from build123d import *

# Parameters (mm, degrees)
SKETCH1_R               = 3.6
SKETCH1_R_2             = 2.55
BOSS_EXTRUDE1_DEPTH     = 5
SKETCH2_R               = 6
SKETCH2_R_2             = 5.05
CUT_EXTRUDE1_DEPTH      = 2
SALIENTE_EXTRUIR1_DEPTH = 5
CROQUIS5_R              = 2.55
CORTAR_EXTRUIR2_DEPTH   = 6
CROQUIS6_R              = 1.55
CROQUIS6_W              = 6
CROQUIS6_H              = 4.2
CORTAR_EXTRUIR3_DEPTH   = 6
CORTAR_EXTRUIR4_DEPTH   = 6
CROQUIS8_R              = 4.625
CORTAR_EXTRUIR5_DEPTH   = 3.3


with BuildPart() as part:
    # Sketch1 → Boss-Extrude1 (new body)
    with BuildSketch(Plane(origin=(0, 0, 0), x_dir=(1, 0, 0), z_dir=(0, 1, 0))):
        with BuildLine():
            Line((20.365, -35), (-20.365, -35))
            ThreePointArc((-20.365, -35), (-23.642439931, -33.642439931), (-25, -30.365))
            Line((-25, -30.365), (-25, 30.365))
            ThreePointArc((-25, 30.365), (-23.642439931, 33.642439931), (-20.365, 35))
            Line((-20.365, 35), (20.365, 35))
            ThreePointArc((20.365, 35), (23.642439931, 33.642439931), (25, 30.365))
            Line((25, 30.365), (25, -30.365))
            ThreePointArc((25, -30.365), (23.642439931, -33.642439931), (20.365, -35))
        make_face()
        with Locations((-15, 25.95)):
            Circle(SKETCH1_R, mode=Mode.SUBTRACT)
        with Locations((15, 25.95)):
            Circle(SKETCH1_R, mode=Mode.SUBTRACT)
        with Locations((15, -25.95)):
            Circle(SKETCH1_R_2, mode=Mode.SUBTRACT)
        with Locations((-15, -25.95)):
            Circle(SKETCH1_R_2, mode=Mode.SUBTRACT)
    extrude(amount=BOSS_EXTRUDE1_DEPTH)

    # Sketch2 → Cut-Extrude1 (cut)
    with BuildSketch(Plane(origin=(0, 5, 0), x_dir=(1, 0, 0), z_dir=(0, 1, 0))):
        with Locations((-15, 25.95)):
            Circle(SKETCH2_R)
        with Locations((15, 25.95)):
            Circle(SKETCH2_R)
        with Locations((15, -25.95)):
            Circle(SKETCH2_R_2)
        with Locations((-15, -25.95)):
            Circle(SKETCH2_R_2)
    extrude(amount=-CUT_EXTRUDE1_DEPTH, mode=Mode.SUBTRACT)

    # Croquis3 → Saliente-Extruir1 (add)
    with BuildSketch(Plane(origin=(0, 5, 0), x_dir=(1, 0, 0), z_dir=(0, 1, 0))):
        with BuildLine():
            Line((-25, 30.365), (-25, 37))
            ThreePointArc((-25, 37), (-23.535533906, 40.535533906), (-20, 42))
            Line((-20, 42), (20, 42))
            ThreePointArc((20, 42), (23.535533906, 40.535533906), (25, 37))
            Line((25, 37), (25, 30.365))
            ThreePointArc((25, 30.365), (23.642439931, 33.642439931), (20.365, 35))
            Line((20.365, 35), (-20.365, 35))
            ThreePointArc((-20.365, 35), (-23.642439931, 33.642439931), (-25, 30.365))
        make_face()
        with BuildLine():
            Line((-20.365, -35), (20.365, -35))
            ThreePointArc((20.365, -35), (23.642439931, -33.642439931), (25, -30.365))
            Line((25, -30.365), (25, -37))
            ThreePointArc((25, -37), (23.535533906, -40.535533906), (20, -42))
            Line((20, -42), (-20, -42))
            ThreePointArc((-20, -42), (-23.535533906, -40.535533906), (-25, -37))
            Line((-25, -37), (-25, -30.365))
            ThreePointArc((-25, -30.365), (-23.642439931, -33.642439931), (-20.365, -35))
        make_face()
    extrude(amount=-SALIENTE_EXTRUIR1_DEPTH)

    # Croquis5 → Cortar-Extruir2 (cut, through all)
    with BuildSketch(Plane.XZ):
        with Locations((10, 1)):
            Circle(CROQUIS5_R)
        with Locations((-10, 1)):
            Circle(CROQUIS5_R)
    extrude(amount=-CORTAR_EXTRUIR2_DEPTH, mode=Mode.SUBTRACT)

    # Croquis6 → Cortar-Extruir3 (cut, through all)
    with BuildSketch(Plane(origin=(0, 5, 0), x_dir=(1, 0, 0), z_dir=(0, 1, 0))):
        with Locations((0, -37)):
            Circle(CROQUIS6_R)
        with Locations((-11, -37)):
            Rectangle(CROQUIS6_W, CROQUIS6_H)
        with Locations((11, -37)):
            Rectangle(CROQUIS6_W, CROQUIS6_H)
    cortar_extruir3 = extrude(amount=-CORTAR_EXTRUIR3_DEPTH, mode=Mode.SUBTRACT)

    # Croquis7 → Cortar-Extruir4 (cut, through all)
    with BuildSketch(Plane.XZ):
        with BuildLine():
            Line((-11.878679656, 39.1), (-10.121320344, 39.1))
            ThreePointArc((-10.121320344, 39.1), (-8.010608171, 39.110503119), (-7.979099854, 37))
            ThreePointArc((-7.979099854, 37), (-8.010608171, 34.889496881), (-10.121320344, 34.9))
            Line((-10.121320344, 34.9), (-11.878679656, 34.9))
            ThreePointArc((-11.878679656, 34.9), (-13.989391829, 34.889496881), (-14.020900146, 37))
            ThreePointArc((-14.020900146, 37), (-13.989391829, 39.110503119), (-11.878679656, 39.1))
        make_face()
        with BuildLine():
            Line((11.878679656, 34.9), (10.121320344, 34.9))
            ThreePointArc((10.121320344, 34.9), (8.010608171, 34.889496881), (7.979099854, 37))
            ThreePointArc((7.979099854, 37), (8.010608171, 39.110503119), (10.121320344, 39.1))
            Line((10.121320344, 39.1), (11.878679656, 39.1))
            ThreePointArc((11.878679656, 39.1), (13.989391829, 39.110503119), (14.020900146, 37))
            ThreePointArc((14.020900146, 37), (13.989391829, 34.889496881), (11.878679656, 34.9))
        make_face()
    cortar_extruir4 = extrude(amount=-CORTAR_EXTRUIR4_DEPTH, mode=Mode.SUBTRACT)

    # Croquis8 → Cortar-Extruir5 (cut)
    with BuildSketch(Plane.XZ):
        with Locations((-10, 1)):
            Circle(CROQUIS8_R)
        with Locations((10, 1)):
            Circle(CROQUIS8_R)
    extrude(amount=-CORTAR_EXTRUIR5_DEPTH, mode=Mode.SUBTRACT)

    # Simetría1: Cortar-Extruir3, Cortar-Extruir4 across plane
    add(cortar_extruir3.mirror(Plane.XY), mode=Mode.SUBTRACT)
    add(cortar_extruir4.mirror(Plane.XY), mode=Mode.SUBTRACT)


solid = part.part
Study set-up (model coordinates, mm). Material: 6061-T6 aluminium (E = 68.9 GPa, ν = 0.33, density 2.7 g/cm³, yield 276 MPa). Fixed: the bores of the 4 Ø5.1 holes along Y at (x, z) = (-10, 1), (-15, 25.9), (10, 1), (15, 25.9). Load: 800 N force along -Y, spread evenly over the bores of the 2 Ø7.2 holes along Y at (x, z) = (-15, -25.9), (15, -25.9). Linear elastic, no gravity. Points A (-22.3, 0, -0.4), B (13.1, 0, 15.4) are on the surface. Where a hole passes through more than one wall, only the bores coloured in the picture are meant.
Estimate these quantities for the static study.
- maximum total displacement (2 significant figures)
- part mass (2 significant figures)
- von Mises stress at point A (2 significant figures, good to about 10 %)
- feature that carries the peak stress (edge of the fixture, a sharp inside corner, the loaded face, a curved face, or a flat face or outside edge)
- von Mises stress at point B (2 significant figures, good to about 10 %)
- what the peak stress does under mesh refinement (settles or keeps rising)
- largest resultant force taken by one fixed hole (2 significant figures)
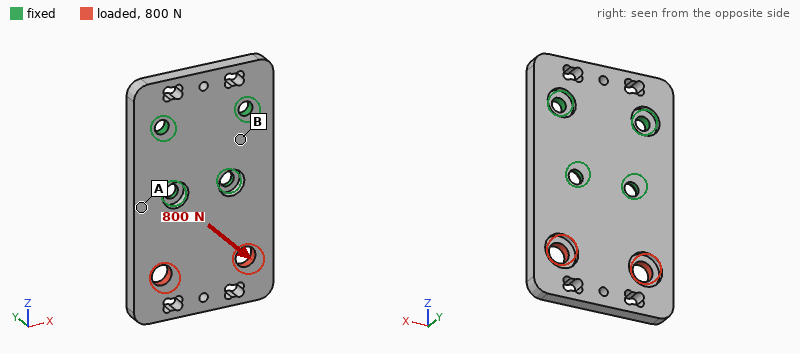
0.42 mm
50 g
86 MPa
edge of the fixture
26 MPa
keeps rising
1.0 kN
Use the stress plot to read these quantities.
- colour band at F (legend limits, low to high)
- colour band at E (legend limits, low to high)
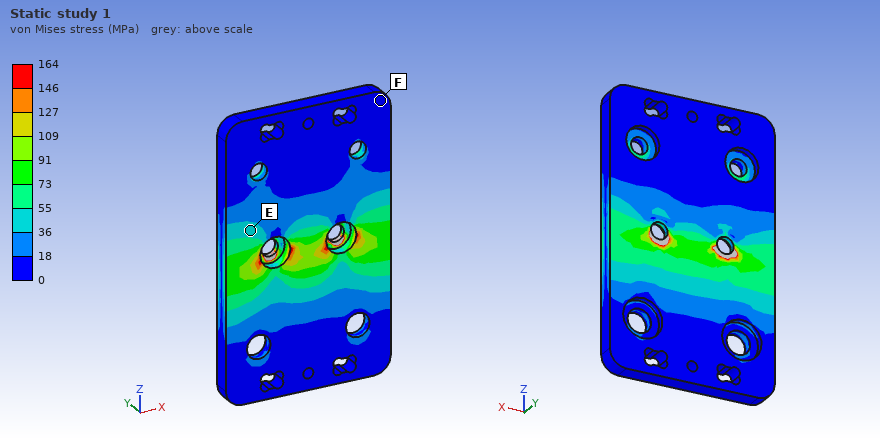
0 to 18 MPa
36 to 55 MPa
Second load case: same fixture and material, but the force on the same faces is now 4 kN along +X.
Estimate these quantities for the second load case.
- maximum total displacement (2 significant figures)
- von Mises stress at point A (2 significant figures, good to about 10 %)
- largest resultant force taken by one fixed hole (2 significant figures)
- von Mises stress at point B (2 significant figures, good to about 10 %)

84 µm
34 MPa
3.2 kN
18 MPa
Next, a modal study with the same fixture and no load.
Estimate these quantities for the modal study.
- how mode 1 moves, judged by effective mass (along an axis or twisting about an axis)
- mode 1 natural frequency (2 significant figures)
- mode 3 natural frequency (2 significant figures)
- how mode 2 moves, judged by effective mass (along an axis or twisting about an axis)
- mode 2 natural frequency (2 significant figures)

along Y
2000 Hz
9400 Hz
twisting about Z
3900 Hz
